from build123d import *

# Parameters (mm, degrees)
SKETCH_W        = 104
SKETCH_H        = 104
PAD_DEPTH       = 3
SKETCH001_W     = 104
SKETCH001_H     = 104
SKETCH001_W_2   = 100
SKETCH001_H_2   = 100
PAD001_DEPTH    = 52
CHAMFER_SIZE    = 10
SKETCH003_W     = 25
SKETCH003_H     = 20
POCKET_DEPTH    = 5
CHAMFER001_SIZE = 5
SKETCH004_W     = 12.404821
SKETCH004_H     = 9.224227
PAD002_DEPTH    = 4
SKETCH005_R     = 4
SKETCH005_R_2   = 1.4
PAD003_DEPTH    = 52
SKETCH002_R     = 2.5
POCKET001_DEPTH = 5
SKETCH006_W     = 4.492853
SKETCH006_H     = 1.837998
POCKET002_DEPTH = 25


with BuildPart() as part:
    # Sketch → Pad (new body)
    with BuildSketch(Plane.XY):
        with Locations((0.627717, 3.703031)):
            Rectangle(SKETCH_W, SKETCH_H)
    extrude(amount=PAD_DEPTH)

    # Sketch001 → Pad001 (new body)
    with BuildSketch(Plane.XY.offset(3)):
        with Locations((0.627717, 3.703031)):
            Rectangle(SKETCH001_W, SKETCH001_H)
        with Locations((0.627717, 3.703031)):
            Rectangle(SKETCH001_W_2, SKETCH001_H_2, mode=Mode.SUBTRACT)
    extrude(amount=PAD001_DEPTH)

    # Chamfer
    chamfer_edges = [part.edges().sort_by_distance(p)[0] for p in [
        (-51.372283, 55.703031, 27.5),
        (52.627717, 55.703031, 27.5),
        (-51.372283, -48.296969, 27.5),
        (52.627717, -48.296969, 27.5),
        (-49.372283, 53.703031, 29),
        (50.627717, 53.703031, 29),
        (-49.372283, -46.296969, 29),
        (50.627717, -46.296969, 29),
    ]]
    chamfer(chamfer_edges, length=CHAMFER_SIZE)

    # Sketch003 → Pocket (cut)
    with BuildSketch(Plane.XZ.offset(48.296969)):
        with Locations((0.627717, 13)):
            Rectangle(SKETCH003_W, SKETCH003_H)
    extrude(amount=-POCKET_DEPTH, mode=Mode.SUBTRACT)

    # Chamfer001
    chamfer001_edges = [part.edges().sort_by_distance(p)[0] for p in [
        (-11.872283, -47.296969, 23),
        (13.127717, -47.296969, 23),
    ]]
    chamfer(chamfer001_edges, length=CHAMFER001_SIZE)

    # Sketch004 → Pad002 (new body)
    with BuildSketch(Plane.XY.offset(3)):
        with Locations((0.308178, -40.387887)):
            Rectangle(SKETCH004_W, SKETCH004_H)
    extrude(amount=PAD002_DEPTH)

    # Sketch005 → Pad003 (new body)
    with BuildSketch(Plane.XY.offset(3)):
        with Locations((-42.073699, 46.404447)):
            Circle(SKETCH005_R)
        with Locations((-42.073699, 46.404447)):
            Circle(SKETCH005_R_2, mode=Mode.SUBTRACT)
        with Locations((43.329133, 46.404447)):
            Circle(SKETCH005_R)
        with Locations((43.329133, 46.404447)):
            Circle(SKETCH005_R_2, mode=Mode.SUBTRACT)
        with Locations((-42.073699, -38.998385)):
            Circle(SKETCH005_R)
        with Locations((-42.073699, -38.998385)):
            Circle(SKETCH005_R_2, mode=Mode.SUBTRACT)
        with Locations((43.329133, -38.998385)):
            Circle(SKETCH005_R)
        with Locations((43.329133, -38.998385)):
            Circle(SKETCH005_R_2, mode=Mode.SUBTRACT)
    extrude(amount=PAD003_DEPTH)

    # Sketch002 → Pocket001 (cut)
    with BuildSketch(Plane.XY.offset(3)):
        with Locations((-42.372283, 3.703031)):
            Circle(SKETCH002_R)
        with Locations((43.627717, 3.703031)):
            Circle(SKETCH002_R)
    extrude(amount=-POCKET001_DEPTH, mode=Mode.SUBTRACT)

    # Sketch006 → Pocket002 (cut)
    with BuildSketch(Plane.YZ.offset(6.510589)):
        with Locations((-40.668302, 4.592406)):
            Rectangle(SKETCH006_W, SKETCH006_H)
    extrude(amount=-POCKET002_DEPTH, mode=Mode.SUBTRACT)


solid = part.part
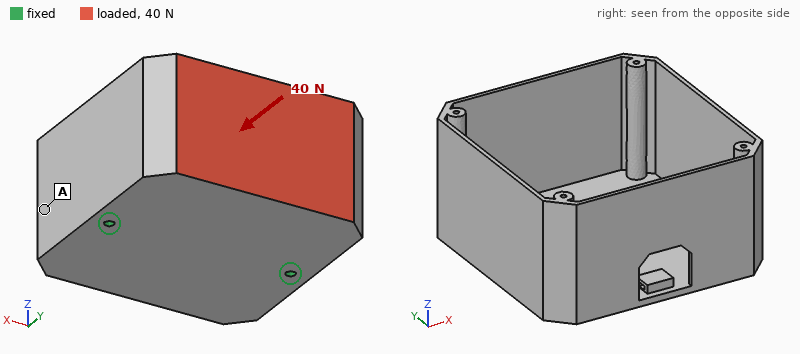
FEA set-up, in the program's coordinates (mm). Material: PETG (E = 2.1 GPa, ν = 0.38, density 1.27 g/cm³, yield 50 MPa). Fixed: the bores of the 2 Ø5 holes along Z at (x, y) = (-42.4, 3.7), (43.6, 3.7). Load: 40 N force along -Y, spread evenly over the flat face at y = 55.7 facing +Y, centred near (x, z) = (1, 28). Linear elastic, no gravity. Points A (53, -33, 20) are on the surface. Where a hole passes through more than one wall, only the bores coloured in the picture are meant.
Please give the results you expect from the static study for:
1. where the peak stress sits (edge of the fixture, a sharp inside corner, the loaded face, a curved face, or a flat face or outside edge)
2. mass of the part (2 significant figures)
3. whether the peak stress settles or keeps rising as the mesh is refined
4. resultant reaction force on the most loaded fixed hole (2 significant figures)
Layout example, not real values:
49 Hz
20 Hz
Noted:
edge of the fixture
100 g
keeps rising
20 N
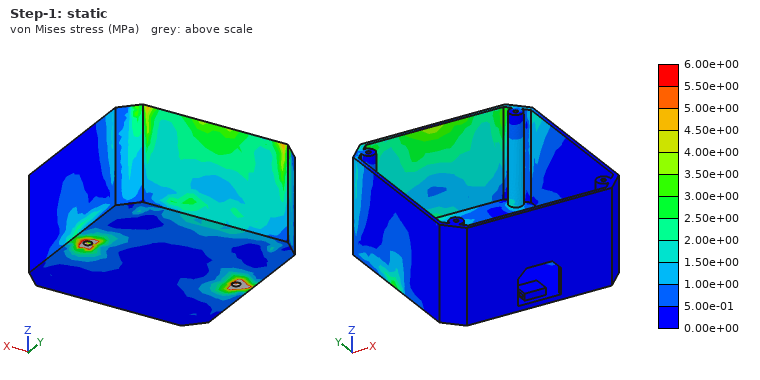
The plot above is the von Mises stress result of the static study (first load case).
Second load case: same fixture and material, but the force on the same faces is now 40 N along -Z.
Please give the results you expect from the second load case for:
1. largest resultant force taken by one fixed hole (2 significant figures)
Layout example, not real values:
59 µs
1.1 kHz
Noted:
20 N
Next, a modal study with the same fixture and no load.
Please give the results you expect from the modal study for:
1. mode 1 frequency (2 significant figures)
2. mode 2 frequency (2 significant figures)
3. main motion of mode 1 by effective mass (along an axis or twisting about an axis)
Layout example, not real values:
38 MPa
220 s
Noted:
110 Hz
150 Hz
along Y
